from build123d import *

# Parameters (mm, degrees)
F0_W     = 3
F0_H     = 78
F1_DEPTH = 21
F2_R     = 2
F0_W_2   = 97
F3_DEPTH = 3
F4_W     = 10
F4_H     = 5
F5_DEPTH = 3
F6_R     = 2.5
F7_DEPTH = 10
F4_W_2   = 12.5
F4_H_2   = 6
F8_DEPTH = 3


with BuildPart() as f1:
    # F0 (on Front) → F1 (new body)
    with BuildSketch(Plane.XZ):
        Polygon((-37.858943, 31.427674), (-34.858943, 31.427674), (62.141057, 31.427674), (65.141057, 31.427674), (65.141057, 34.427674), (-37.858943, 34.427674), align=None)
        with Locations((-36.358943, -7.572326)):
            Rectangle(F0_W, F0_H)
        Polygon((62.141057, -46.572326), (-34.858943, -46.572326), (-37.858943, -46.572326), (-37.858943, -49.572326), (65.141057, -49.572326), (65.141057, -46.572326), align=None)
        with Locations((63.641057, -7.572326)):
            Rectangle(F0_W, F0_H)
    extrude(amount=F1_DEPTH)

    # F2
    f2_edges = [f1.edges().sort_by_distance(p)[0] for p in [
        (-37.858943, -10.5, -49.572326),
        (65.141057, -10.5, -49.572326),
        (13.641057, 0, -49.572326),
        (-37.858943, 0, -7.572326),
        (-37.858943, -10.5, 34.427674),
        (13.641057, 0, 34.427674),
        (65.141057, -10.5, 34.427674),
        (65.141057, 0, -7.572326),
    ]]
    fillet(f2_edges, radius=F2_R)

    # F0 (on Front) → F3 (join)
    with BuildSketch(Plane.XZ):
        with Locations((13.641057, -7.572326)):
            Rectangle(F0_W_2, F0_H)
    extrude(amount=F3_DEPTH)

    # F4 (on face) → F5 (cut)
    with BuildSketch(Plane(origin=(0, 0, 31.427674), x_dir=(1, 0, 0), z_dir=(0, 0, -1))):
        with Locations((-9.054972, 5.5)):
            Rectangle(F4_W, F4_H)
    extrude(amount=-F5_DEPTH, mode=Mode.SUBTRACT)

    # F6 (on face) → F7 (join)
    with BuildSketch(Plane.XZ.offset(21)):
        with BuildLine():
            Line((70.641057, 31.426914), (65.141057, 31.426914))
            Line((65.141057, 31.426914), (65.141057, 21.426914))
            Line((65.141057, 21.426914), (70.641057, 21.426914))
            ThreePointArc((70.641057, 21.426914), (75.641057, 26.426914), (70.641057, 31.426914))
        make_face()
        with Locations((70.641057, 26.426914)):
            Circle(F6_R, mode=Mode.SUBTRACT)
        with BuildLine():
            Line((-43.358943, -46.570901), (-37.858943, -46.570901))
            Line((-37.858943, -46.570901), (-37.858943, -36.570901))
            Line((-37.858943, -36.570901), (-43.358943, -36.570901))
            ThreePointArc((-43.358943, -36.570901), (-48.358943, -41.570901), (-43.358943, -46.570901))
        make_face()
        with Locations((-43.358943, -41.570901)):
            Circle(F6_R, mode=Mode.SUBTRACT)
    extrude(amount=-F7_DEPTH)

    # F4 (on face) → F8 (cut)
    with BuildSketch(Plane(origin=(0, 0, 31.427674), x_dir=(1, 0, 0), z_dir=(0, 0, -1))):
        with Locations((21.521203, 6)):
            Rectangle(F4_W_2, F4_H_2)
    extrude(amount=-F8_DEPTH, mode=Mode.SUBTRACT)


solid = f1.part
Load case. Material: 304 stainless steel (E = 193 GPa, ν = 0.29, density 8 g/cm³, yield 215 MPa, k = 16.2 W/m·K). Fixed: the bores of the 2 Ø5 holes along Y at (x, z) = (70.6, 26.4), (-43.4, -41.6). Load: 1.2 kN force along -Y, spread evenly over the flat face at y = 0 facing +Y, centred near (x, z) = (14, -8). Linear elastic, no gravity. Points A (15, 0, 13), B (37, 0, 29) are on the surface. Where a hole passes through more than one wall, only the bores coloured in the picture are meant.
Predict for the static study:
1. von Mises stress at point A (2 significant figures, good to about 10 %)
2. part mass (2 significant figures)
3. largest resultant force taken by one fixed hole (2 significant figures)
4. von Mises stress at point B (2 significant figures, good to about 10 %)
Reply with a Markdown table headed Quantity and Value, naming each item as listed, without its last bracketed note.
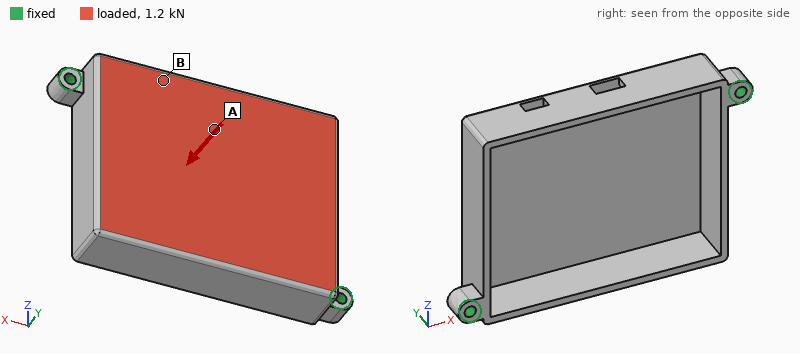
| Quantity | Value |
|---|---|
| von Mises stress at point A | 22 MPa |
| part mass | 370 g |
| largest resultant force taken by one fixed hole | 1.2 kN |
| von Mises stress at point B | 11 MPa |
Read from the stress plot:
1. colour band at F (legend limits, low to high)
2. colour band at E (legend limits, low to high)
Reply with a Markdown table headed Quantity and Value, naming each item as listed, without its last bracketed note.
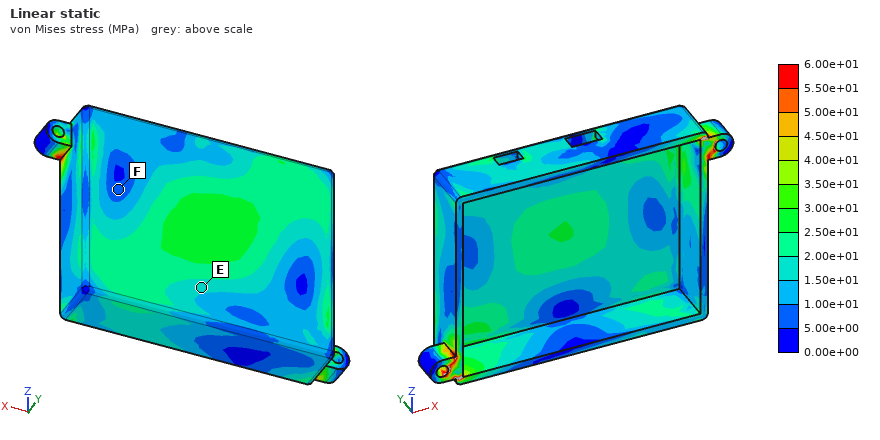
| Quantity | Value |
|---|---|
| colour band at F | 5.00e+00 to 1.00e+01 MPa |
| colour band at E | 1.50e+01 to 2.00e+01 MPa |
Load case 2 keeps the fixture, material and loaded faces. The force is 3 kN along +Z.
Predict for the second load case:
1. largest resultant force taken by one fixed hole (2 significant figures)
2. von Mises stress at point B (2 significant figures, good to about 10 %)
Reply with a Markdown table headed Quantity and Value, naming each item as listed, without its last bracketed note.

| Quantity | Value |
|---|---|
| largest resultant force taken by one fixed hole | 1.5 kN |
| von Mises stress at point B | 16 MPa |
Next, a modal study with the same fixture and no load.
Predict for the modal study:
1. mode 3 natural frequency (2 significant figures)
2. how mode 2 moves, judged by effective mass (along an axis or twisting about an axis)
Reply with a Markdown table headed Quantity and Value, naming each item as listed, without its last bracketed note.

| Quantity | Value |
|---|---|
| mode 3 natural frequency | 2700 Hz |
| how mode 2 moves, judged by effective mass | along Y |
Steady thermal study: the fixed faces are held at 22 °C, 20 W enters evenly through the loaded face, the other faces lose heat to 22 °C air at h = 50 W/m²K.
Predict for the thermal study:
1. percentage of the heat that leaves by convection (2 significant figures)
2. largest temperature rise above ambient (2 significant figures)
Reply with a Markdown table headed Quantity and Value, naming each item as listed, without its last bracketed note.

| Quantity | Value |
|---|---|
| percentage of the heat that leaves by convection | 90 % |
| largest temperature rise above ambient | 31 K |
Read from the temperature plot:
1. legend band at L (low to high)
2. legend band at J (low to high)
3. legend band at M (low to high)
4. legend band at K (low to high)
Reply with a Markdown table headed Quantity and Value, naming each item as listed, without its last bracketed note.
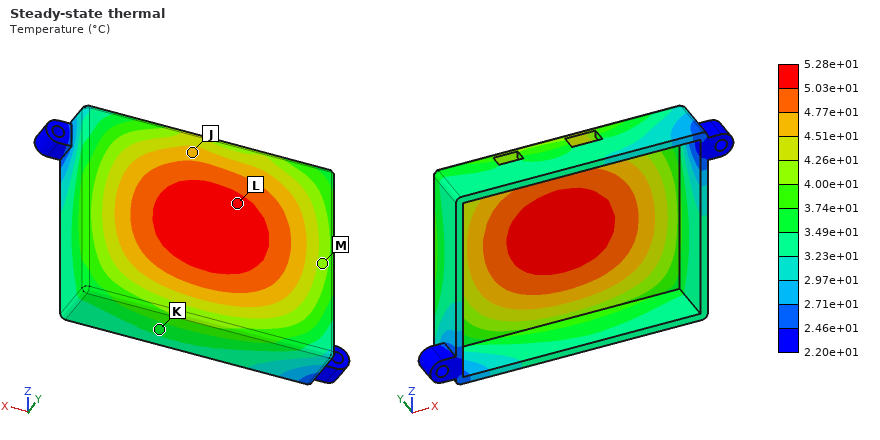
| Quantity | Value |
|---|---|
| legend band at L | 5.03e+01 to 5.28e+01 °C |
| legend band at J | 4.51e+01 to 4.77e+01 °C |
| legend band at M | 4.00e+01 to 4.26e+01 °C |
| legend band at K | 3.49e+01 to 3.74e+01 °C |
